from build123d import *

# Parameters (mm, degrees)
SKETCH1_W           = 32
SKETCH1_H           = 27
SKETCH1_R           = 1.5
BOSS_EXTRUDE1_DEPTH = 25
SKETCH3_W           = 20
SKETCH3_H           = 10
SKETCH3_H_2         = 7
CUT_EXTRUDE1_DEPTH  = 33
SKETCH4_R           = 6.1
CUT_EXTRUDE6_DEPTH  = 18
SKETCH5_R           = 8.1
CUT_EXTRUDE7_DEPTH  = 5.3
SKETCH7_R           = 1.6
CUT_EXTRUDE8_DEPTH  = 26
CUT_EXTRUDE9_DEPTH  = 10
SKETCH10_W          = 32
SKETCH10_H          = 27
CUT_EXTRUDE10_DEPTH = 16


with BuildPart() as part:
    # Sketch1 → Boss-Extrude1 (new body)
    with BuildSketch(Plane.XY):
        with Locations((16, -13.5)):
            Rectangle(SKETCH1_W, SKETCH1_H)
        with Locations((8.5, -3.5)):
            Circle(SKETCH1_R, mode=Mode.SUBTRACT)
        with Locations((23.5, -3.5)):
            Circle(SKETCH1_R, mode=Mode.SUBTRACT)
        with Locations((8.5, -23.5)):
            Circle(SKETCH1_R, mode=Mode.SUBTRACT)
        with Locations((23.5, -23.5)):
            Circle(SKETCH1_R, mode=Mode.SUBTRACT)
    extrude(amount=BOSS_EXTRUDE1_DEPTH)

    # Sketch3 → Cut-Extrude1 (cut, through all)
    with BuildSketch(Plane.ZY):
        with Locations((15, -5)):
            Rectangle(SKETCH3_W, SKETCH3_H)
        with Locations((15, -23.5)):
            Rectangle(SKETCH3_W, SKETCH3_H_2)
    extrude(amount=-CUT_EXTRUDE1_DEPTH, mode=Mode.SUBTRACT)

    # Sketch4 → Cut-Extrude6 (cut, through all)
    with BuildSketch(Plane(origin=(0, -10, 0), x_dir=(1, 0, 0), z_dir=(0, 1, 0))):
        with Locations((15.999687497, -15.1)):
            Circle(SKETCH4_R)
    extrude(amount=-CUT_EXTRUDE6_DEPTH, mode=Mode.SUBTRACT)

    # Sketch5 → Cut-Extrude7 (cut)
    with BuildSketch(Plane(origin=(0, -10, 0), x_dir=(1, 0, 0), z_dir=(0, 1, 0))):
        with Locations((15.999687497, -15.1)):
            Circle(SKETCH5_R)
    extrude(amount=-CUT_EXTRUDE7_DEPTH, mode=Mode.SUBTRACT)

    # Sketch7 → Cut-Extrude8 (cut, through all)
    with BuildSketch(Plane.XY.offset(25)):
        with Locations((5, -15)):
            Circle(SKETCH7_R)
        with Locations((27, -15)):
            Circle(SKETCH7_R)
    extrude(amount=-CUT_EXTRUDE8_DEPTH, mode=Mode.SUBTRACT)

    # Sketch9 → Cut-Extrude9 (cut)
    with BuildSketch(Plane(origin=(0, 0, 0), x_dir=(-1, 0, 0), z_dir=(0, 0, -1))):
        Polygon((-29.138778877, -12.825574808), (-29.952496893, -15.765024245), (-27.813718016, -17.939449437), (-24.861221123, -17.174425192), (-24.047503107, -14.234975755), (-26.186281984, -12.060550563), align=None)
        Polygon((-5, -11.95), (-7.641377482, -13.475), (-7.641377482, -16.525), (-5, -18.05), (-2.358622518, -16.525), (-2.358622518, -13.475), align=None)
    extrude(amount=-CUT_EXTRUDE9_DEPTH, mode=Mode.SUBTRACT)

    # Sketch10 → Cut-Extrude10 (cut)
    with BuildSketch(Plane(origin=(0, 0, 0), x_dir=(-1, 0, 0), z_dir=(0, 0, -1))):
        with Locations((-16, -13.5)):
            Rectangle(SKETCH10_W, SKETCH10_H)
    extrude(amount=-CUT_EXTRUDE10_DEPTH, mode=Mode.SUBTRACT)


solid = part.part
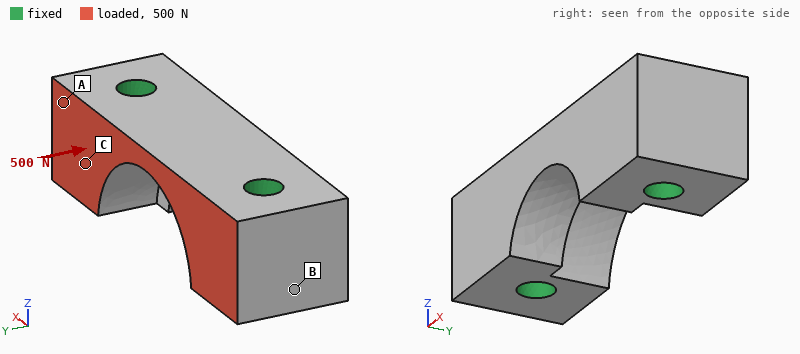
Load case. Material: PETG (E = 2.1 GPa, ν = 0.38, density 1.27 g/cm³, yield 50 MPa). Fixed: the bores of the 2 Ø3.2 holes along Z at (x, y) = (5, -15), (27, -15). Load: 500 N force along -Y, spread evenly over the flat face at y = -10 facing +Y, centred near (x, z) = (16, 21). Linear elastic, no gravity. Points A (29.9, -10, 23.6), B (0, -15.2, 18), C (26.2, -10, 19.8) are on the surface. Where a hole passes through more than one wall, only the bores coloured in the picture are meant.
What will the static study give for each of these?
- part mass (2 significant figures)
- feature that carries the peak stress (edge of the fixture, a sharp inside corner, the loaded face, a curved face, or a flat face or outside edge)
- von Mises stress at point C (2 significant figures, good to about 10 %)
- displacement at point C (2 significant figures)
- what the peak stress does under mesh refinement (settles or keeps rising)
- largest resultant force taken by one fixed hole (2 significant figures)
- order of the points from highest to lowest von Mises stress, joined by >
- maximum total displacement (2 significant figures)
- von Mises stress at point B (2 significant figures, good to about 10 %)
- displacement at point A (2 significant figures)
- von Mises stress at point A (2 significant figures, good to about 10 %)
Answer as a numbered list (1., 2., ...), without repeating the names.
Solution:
1. 2.6 g
2. edge of the fixture
3. 4.5 MPa
4. 6.7 µm
5. keeps rising
6. 250 N
7. C > A > B
8. 31 µm
9. 1.4 MPa
10. 7.4 µm
11. 2.9 MPa
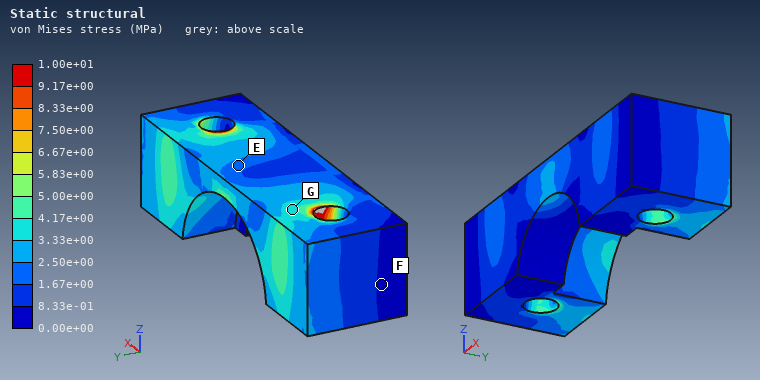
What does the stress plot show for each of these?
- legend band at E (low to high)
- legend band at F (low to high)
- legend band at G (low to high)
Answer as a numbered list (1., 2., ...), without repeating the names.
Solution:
1. 1.67e+00 to 2.50e+00 MPa
2. 0.00e+00 to 8.33e-01 MPa
3. 3.33e+00 to 4.17e+00 MPa
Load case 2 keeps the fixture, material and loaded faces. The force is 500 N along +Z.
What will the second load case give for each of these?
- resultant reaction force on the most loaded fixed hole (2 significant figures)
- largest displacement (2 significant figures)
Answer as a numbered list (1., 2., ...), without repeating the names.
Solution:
1. 250 N
2. 0.10 mm
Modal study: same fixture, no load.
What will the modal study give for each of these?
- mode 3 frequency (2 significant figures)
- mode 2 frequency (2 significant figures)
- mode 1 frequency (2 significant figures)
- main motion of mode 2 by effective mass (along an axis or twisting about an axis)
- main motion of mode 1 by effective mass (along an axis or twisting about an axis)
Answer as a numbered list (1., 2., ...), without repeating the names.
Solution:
1. 21 kHz
2. 17 kHz
3. 14 kHz
4. along Z
5. along Y
